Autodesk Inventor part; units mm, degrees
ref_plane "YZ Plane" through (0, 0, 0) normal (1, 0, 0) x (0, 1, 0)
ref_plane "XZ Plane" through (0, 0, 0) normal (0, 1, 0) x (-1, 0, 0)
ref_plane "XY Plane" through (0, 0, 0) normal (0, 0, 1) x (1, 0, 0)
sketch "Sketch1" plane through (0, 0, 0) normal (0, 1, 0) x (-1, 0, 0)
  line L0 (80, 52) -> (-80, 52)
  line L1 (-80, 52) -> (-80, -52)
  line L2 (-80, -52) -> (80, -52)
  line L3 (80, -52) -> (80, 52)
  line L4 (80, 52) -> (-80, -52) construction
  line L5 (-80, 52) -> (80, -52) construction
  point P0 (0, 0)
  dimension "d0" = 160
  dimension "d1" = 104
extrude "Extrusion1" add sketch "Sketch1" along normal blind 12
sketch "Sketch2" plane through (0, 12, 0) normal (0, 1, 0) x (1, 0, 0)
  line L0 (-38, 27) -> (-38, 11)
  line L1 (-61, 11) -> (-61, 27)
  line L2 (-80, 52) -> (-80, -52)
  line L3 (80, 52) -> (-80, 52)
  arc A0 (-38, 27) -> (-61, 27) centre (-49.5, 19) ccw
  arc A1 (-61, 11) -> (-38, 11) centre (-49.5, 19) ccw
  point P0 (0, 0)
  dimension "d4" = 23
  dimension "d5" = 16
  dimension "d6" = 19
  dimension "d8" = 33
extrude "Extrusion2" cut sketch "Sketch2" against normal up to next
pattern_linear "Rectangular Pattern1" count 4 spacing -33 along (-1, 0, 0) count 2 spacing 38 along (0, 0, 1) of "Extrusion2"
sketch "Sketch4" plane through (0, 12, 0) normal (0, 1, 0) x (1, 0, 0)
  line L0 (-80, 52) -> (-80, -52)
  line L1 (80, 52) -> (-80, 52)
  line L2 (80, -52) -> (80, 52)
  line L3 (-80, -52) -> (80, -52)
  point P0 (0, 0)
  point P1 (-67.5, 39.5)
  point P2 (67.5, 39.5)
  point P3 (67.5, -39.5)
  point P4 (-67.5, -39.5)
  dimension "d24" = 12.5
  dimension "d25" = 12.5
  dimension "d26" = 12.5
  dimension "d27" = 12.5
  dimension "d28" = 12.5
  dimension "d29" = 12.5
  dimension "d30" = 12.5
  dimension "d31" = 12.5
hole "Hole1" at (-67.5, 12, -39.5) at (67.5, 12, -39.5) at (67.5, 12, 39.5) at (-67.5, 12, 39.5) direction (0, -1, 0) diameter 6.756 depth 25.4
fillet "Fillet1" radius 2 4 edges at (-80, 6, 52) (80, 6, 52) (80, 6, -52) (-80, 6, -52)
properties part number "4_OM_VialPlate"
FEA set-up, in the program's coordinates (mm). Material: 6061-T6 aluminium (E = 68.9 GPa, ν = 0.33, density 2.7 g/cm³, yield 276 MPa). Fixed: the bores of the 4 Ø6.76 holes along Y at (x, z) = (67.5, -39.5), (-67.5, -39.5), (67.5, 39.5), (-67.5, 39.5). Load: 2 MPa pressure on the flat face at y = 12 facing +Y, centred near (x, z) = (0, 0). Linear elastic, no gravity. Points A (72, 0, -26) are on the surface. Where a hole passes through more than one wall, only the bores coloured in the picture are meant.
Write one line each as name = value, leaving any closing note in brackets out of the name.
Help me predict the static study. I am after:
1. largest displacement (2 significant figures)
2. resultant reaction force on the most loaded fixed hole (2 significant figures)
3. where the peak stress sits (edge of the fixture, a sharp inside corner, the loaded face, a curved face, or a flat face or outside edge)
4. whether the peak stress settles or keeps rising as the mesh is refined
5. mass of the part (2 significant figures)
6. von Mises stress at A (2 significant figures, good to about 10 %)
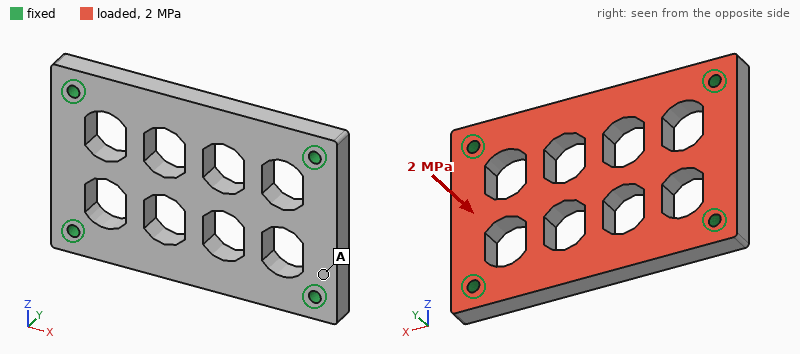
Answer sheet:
largest displacement = 0.29 mm
resultant reaction force on the most loaded fixed hole = 6.0 kN
where the peak stress sits = edge of the fixture
whether the peak stress settles or keeps rising as the mesh is refined = keeps rising
mass of the part = 390 g
von Mises stress at A = 32 MPa
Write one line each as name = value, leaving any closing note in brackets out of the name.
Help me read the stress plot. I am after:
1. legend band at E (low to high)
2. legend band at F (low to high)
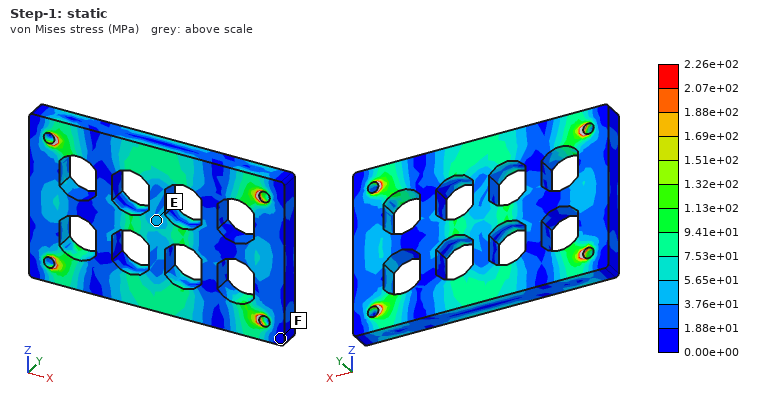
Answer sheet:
legend band at E = 3.76e+01 to 5.65e+01 MPa
legend band at F = 0.00e+00 to 1.88e+01 MPa
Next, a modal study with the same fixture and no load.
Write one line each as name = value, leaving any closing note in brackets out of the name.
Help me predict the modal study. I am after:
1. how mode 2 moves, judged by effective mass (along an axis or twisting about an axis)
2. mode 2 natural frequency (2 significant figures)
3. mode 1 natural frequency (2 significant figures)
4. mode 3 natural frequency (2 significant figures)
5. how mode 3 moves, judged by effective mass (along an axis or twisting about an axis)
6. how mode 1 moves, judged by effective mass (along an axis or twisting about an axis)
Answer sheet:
how mode 2 moves, judged by effective mass = twisting about X
mode 2 natural frequency = 3700 Hz
mode 1 natural frequency = 2700 Hz
mode 3 natural frequency = 5800 Hz
how mode 3 moves, judged by effective mass = along Z
how mode 1 moves, judged by effective mass = along Y
